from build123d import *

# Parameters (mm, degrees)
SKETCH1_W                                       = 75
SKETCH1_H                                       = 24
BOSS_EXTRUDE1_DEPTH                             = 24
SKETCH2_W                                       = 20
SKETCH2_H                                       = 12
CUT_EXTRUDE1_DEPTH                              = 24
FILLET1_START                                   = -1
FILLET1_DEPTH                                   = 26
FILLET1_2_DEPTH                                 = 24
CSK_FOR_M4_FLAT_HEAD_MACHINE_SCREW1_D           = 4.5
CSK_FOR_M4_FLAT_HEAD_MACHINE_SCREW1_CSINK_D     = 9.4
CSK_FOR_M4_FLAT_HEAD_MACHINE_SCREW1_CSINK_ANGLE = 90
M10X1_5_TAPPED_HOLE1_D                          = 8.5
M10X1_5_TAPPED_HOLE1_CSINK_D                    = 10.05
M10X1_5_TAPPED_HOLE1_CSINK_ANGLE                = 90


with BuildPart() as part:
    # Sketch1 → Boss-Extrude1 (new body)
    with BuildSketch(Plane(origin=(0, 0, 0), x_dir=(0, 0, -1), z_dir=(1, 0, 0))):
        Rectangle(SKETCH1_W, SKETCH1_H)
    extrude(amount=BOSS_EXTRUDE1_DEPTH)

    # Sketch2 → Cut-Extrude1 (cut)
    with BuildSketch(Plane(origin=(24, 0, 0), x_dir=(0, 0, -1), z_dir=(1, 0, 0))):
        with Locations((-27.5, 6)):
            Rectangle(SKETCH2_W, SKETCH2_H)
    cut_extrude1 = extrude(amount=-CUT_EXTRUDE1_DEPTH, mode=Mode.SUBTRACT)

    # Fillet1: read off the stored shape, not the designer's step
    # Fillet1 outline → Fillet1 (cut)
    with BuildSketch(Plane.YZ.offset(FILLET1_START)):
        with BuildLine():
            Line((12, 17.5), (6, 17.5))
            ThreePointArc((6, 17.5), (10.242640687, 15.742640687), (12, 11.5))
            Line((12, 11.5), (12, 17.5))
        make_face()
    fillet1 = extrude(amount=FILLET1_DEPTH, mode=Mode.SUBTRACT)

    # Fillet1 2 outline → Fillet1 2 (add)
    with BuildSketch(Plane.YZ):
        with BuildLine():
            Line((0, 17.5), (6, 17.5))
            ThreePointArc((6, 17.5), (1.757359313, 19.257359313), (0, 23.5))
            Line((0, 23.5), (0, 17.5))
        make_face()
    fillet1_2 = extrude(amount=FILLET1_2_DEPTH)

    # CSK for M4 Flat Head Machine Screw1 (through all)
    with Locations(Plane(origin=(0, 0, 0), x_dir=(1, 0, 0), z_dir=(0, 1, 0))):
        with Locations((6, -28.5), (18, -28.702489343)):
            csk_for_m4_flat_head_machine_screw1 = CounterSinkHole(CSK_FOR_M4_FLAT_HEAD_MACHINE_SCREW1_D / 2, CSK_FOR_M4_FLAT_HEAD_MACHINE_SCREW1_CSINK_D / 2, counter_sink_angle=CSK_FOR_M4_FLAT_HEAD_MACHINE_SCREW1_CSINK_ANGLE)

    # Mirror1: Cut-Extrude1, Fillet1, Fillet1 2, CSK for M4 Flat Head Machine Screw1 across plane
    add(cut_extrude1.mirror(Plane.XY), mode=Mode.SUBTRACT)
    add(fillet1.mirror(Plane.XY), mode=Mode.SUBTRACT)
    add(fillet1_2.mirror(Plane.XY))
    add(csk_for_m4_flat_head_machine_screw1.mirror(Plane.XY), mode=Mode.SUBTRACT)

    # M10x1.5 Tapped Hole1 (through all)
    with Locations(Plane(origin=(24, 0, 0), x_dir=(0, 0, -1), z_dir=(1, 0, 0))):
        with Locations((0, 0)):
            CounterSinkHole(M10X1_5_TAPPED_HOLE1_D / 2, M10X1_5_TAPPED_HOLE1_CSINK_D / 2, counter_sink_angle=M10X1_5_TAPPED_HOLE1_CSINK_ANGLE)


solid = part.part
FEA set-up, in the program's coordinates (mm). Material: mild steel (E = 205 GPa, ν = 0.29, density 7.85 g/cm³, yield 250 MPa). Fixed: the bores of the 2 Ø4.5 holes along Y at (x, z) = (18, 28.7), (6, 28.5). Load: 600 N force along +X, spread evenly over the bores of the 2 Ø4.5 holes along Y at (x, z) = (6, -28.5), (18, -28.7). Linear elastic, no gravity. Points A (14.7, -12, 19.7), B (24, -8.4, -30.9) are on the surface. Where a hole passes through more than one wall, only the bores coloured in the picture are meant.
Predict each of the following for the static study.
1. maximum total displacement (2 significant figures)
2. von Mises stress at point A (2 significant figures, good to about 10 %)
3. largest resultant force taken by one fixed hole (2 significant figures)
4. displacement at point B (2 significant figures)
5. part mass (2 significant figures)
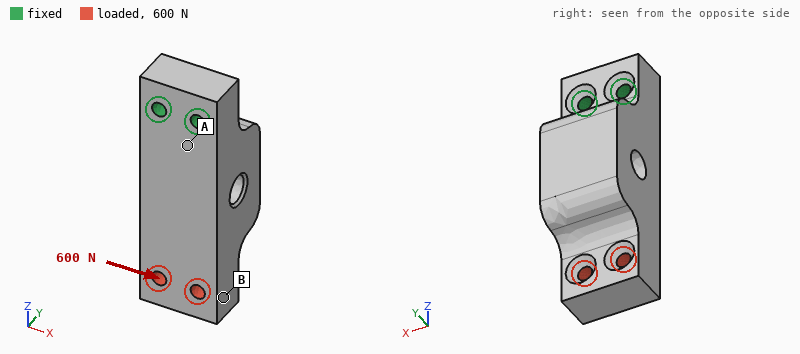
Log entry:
19 µm
15 MPa
2.3 kN
17 µm
230 g
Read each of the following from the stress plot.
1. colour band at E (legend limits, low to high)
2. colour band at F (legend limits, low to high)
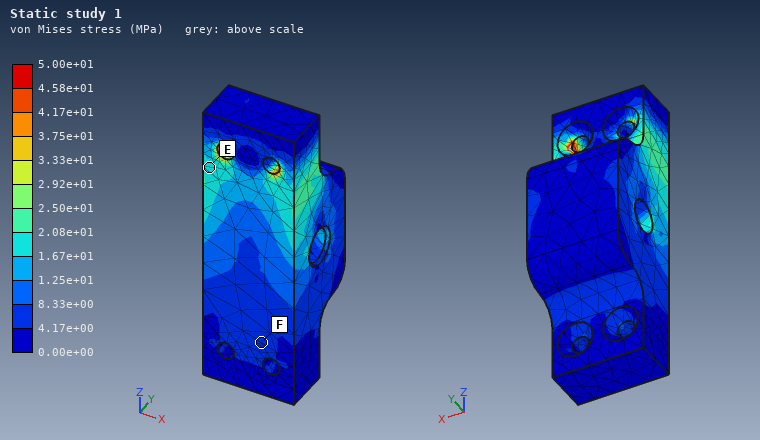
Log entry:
1.67e+01 to 2.08e+01 MPa
4.17e+00 to 8.33e+00 MPa
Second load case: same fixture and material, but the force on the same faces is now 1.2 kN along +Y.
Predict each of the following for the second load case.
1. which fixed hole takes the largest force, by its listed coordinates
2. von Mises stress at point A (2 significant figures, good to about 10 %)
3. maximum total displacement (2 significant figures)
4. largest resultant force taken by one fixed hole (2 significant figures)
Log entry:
(6, 28.5)
84 MPa
92 µm
650 N
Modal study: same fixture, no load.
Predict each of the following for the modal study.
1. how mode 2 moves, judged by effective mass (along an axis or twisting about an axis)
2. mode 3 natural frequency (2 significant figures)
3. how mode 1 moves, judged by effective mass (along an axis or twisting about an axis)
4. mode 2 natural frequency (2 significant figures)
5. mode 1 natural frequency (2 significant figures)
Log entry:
along X
8600 Hz
along Y
3800 Hz
2300 Hz
